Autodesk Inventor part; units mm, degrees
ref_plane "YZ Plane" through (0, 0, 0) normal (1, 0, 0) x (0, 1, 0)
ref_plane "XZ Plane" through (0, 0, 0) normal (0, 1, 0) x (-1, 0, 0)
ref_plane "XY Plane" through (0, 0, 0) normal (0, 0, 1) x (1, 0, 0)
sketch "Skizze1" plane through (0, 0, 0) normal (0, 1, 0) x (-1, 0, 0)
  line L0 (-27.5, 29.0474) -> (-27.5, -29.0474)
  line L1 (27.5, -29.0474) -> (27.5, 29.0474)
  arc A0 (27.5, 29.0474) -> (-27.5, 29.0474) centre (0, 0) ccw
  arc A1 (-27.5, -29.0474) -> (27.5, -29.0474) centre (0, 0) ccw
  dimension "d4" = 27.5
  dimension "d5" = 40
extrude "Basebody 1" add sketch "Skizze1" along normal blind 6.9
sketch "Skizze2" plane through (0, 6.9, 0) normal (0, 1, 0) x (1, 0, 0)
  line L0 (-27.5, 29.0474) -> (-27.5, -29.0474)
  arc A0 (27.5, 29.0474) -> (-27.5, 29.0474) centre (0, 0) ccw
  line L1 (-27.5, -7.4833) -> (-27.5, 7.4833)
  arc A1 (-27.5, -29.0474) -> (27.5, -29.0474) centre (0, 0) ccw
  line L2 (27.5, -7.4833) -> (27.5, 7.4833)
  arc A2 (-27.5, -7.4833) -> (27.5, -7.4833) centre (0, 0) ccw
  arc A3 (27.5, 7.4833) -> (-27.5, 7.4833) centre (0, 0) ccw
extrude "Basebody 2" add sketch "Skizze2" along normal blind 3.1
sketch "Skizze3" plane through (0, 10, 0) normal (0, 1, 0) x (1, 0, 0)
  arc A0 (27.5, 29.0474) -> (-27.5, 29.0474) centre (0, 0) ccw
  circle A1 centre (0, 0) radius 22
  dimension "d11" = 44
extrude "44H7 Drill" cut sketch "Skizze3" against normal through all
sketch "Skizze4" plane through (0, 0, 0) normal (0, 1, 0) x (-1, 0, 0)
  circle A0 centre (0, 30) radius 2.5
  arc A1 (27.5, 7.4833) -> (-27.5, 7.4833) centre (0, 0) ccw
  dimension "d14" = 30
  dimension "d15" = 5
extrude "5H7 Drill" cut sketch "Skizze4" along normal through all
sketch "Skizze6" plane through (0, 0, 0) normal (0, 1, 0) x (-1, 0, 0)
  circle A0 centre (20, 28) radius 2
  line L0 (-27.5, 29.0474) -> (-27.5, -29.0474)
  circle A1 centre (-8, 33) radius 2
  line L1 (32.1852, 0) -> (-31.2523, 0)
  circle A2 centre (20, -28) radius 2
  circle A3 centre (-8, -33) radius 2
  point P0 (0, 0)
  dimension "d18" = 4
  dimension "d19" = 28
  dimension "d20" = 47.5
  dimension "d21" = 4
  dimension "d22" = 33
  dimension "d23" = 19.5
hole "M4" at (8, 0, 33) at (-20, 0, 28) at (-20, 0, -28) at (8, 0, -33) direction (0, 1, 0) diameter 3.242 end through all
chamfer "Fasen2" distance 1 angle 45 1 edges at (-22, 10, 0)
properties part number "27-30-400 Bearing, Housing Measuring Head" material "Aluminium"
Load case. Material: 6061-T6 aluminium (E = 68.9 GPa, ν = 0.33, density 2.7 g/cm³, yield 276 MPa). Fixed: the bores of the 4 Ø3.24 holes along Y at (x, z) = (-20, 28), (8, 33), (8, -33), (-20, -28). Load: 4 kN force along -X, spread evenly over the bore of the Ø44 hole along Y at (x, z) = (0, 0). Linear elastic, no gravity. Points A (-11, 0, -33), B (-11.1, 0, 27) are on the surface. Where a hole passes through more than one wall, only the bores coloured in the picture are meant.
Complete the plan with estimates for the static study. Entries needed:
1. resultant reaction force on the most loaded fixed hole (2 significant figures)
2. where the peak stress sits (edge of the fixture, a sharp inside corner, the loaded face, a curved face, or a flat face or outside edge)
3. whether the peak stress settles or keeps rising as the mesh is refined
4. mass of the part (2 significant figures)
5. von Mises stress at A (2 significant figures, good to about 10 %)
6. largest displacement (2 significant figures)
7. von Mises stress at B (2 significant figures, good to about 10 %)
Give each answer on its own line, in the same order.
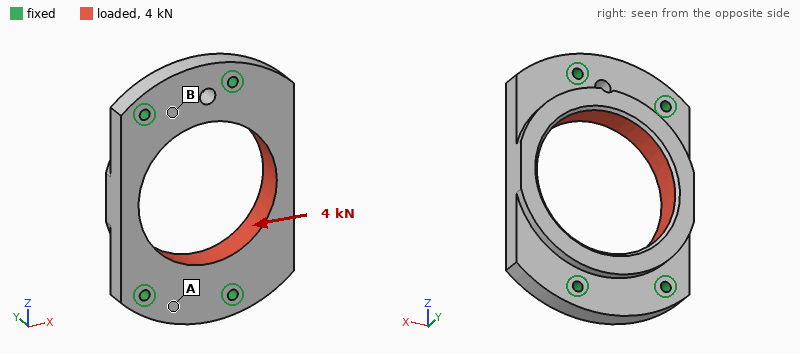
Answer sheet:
1.1 kN
edge of the fixture
keeps rising
54 g
4.9 MPa
14 µm
12 MPa
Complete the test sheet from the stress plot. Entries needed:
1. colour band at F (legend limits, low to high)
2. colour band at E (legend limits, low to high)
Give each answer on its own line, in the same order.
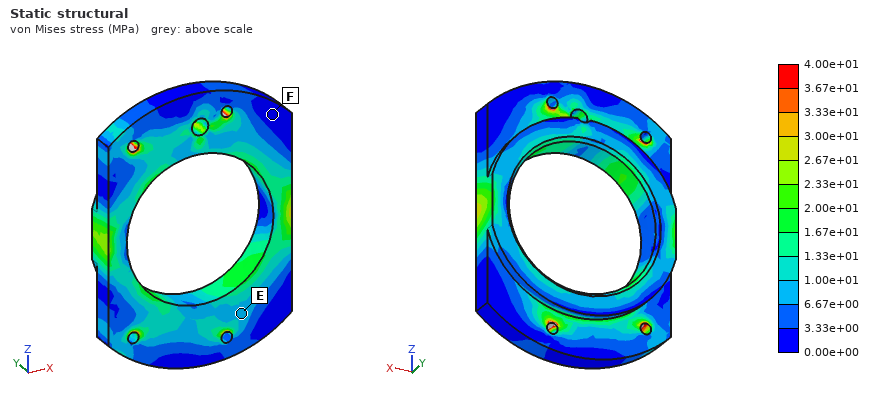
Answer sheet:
0.00e+00 to 3.33e+00 MPa
6.67e+00 to 1.00e+01 MPa
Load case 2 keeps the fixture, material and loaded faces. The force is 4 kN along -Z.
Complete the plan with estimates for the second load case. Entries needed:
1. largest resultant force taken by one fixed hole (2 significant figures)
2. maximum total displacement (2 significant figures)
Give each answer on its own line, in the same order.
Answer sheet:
1.3 kN
8.5 µm
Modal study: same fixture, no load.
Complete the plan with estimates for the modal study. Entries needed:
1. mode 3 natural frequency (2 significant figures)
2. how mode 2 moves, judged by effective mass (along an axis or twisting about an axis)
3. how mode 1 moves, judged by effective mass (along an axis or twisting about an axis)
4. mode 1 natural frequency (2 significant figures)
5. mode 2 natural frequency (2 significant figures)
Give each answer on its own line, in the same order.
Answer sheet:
14 kHz
along Y
along Y
6800 Hz
13 kHz
